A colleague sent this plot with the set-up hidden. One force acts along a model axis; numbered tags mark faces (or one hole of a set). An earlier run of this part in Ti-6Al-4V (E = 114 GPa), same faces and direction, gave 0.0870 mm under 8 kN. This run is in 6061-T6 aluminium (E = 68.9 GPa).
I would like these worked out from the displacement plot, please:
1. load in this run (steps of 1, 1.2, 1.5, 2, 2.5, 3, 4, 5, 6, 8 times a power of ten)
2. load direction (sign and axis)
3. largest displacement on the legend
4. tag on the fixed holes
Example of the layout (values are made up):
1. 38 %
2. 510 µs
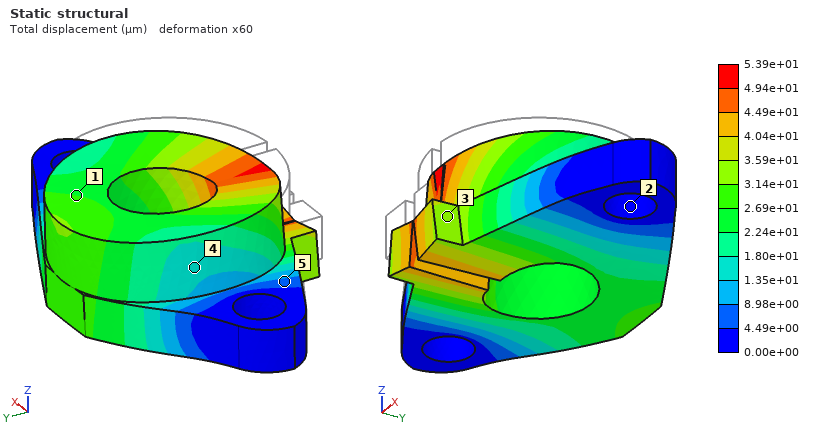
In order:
1. 3 kN
2. -Z
3. 5.39e+01 µm
4. 2
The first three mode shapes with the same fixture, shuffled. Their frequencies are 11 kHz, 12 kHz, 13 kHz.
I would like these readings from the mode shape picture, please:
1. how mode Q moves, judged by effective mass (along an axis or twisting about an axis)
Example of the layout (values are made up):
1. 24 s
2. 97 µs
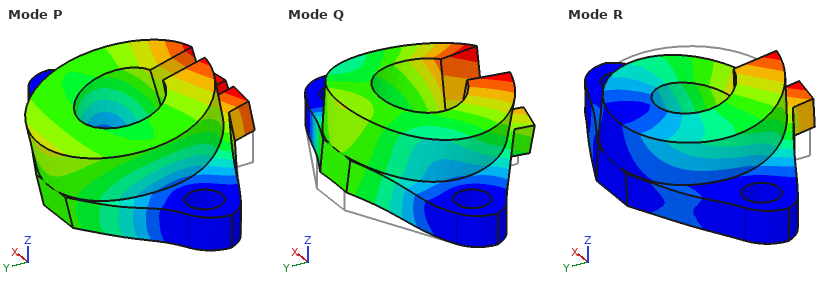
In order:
1. along Z
